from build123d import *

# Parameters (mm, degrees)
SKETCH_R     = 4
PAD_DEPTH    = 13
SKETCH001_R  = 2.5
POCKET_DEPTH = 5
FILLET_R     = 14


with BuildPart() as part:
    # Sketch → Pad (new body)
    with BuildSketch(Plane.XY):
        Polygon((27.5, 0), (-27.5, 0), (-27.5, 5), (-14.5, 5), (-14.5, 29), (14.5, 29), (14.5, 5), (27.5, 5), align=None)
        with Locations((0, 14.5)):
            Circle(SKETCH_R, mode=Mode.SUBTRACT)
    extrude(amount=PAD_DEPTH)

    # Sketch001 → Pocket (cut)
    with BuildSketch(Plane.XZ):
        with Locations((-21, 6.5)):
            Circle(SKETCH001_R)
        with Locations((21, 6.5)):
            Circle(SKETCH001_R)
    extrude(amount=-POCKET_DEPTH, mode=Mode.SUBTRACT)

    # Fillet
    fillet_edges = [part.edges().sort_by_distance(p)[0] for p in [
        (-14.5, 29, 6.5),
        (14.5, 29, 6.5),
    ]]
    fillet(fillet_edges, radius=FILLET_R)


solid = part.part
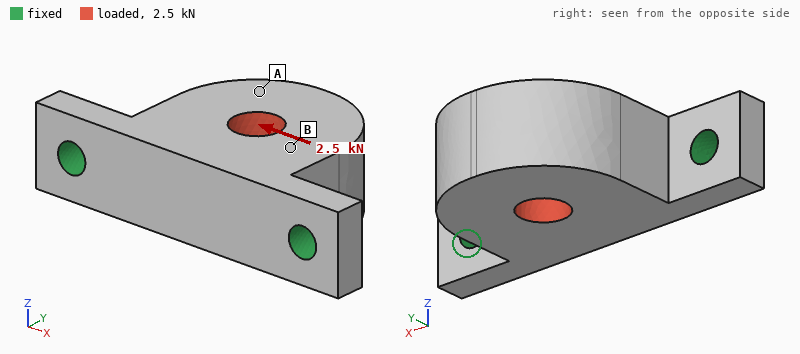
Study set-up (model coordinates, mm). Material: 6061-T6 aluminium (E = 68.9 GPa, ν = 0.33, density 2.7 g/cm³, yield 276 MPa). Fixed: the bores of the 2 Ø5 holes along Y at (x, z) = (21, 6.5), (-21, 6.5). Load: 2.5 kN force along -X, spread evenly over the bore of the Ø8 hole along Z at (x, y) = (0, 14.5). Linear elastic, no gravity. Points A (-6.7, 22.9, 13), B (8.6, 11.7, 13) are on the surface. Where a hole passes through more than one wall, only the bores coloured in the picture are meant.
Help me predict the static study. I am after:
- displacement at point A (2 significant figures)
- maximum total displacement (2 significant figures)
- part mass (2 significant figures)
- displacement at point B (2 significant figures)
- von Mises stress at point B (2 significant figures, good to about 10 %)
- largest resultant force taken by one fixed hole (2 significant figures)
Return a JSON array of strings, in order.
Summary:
["16 µm", "18 µm", "29 g", "8.9 µm", "15 MPa", "1.5 kN"]
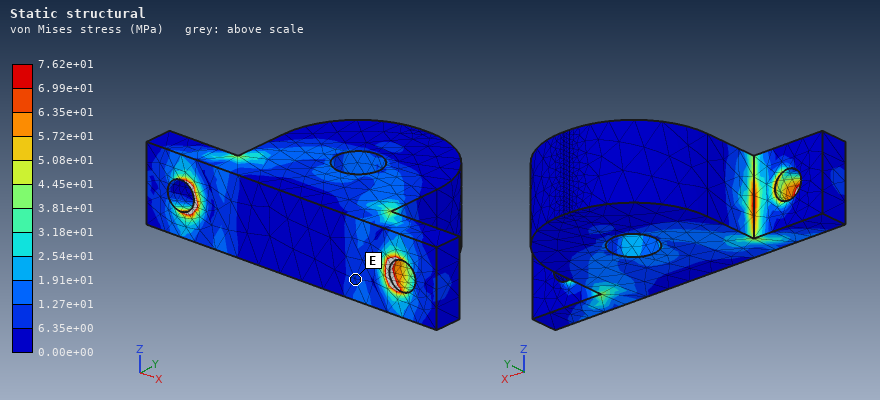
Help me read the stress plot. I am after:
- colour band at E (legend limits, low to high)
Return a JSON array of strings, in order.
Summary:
["6.35e+00 to 1.27e+01 MPa"]
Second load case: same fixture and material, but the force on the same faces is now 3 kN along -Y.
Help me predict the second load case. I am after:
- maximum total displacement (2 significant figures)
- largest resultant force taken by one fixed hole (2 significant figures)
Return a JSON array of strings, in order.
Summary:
["19 µm", "1.7 kN"]
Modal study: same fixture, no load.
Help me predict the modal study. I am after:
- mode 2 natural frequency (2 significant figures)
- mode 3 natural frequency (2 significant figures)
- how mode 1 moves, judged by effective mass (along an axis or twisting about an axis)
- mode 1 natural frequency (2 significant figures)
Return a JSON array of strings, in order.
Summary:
["14 kHz", "14 kHz", "along Z", "4300 Hz"]
